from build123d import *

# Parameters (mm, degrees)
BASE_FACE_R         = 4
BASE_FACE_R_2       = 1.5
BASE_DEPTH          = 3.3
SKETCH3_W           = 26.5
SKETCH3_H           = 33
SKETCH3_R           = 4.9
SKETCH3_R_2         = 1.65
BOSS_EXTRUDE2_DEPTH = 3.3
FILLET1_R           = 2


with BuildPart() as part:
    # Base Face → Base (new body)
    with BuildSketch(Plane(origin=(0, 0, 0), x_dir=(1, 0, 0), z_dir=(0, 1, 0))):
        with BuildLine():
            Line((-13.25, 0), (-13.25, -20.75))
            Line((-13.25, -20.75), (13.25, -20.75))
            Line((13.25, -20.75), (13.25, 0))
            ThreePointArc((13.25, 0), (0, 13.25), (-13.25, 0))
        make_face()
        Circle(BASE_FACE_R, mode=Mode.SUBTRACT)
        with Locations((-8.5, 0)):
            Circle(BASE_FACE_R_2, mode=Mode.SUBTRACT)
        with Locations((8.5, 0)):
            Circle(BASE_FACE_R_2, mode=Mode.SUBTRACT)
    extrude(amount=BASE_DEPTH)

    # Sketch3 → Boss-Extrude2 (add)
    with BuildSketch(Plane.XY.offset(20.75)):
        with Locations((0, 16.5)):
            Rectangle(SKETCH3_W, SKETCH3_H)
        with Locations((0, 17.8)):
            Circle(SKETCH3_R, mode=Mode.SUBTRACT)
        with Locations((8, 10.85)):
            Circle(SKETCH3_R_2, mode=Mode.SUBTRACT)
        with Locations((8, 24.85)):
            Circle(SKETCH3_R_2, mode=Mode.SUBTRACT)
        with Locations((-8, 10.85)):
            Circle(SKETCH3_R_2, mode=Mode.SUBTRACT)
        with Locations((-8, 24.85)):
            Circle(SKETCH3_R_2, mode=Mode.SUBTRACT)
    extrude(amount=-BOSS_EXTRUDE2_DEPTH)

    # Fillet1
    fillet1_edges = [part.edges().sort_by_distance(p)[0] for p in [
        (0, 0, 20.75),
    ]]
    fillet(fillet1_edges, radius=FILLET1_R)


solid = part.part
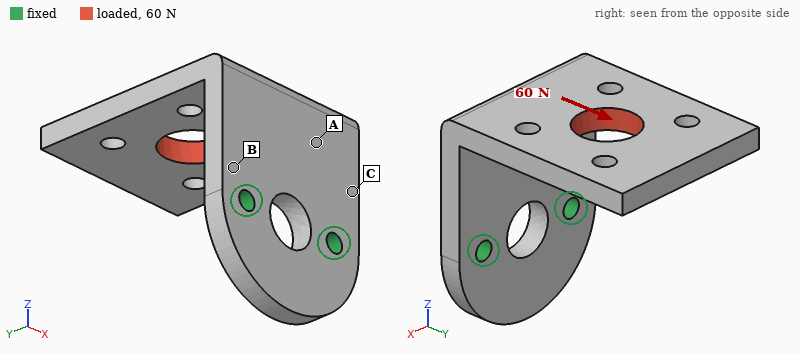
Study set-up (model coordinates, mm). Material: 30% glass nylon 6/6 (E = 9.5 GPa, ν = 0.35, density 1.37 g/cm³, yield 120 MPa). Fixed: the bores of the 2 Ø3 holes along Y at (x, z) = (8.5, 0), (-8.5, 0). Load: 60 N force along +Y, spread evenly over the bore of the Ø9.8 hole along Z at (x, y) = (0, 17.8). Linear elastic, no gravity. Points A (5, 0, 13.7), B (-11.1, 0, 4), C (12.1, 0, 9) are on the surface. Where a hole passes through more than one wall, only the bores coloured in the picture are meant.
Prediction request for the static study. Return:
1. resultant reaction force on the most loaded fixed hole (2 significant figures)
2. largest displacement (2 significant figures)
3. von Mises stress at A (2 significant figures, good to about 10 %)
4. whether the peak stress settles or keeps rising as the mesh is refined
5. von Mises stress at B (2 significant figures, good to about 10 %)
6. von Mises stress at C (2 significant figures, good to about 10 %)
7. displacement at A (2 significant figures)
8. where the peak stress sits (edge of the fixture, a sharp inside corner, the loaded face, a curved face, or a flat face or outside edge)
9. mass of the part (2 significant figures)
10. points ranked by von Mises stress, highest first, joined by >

30 N
0.54 mm
6.2 MPa
keeps rising
22 MPa
15 MPa
0.13 mm
edge of the fixture
6.5 g
B > C > A
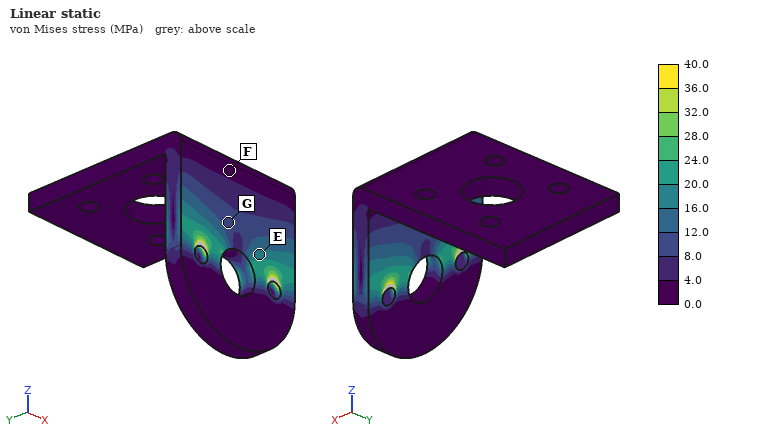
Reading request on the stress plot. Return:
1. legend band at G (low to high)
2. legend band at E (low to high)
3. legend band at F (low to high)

8.0 to 12.0 MPa
16.0 to 20.0 MPa
0.0 to 4.0 MPa
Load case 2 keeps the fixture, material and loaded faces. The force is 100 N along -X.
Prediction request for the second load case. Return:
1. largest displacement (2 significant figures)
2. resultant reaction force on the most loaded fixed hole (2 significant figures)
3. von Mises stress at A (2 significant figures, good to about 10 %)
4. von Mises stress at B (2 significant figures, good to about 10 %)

0.56 mm
140 N
17 MPa
25 MPa
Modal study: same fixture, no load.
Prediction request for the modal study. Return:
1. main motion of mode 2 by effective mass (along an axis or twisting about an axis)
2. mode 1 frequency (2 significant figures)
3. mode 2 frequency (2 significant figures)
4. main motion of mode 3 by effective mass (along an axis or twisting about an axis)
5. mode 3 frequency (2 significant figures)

along X
730 Hz
1400 Hz
along Y
2200 Hz
